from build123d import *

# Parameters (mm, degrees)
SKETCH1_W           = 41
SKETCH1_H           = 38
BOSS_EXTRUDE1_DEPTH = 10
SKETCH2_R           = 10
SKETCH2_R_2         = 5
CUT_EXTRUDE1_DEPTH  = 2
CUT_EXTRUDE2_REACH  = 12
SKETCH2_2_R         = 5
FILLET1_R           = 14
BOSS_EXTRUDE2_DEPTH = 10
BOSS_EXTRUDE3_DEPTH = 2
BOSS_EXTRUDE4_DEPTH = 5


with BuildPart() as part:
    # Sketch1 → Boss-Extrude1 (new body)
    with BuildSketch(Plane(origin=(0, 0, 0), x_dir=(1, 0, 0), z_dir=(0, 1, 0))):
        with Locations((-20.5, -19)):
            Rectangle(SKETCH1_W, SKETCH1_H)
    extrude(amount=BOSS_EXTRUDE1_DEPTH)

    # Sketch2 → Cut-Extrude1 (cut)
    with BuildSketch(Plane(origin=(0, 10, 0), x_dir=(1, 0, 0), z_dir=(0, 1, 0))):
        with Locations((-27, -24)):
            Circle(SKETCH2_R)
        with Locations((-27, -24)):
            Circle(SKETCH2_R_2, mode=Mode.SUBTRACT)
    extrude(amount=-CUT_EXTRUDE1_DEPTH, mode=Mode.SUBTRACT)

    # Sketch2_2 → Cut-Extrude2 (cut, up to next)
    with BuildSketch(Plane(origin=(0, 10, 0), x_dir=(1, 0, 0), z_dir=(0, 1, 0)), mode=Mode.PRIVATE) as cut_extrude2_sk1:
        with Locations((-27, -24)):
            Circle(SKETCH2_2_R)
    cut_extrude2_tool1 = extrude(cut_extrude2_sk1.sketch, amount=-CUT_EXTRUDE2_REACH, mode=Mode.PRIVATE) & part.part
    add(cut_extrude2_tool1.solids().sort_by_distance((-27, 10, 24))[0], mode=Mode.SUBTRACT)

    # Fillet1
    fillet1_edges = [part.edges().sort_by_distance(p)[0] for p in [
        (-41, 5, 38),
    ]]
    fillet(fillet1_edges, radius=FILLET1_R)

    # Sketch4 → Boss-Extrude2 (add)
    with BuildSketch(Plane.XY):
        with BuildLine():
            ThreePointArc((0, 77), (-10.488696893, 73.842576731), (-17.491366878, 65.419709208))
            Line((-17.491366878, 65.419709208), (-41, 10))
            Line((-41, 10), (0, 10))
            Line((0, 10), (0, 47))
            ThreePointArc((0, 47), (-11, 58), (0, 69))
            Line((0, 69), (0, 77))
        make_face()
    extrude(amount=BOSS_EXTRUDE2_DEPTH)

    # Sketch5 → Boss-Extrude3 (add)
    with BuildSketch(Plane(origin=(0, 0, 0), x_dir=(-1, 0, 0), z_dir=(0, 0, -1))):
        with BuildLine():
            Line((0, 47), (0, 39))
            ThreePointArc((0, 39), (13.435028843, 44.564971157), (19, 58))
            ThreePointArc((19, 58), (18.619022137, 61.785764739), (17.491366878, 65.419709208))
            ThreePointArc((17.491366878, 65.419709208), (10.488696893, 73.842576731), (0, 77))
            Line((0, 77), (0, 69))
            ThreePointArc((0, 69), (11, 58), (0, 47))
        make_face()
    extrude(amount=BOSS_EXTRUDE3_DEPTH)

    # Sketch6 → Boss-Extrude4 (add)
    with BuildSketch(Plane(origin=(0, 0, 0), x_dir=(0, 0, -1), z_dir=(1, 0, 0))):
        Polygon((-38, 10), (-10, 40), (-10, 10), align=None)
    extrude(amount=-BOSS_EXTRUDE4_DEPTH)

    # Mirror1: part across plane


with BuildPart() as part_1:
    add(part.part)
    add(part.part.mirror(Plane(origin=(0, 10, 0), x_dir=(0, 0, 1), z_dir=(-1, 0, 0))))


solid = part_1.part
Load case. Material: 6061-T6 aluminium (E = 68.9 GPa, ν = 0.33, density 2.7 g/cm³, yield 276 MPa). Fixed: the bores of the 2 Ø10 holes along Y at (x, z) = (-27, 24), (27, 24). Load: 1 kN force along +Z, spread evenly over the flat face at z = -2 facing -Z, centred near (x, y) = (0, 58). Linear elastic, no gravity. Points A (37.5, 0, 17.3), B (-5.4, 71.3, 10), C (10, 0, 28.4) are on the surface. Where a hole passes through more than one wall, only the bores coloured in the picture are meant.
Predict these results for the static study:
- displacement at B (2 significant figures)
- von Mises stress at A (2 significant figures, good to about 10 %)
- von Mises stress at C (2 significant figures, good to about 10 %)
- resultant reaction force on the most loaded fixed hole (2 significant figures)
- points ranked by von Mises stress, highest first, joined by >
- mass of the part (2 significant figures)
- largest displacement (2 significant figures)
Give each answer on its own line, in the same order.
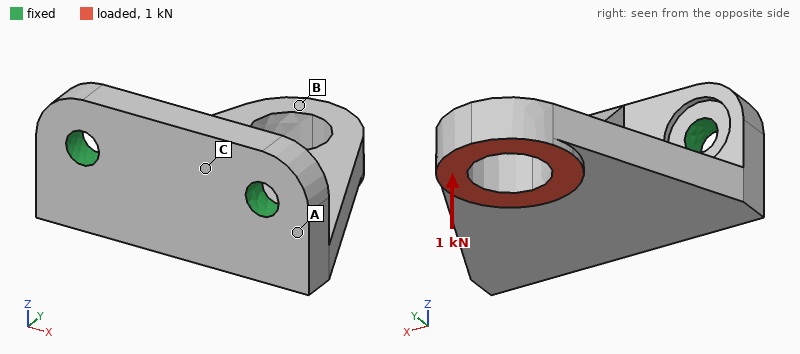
0.18 mm
25 MPa
16 MPa
600 N
A > C > B
180 g
0.21 mm
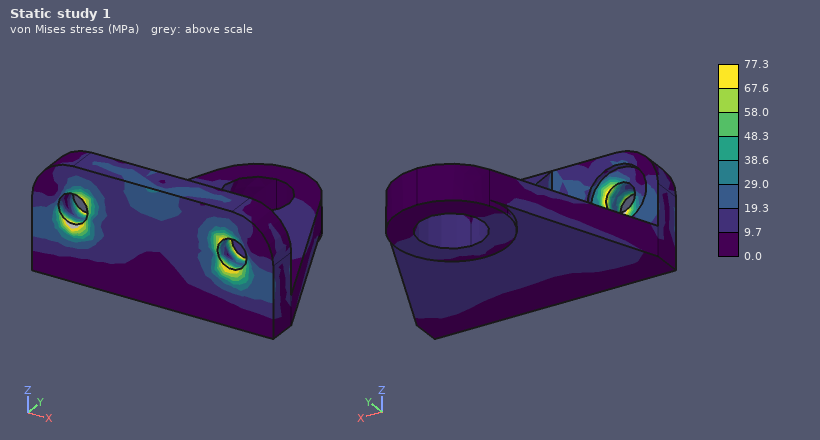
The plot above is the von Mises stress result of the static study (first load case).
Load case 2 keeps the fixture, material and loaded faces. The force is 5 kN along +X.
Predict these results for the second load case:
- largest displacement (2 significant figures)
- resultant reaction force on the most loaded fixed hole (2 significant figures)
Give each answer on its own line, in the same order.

0.14 mm
5.8 kN
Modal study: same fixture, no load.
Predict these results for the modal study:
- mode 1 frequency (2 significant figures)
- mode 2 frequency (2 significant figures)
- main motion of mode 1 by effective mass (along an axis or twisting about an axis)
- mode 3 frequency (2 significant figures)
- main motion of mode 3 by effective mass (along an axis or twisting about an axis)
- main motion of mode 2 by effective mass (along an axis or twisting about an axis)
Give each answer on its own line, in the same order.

2200 Hz
5000 Hz
along Z
6500 Hz
along Y
along X
